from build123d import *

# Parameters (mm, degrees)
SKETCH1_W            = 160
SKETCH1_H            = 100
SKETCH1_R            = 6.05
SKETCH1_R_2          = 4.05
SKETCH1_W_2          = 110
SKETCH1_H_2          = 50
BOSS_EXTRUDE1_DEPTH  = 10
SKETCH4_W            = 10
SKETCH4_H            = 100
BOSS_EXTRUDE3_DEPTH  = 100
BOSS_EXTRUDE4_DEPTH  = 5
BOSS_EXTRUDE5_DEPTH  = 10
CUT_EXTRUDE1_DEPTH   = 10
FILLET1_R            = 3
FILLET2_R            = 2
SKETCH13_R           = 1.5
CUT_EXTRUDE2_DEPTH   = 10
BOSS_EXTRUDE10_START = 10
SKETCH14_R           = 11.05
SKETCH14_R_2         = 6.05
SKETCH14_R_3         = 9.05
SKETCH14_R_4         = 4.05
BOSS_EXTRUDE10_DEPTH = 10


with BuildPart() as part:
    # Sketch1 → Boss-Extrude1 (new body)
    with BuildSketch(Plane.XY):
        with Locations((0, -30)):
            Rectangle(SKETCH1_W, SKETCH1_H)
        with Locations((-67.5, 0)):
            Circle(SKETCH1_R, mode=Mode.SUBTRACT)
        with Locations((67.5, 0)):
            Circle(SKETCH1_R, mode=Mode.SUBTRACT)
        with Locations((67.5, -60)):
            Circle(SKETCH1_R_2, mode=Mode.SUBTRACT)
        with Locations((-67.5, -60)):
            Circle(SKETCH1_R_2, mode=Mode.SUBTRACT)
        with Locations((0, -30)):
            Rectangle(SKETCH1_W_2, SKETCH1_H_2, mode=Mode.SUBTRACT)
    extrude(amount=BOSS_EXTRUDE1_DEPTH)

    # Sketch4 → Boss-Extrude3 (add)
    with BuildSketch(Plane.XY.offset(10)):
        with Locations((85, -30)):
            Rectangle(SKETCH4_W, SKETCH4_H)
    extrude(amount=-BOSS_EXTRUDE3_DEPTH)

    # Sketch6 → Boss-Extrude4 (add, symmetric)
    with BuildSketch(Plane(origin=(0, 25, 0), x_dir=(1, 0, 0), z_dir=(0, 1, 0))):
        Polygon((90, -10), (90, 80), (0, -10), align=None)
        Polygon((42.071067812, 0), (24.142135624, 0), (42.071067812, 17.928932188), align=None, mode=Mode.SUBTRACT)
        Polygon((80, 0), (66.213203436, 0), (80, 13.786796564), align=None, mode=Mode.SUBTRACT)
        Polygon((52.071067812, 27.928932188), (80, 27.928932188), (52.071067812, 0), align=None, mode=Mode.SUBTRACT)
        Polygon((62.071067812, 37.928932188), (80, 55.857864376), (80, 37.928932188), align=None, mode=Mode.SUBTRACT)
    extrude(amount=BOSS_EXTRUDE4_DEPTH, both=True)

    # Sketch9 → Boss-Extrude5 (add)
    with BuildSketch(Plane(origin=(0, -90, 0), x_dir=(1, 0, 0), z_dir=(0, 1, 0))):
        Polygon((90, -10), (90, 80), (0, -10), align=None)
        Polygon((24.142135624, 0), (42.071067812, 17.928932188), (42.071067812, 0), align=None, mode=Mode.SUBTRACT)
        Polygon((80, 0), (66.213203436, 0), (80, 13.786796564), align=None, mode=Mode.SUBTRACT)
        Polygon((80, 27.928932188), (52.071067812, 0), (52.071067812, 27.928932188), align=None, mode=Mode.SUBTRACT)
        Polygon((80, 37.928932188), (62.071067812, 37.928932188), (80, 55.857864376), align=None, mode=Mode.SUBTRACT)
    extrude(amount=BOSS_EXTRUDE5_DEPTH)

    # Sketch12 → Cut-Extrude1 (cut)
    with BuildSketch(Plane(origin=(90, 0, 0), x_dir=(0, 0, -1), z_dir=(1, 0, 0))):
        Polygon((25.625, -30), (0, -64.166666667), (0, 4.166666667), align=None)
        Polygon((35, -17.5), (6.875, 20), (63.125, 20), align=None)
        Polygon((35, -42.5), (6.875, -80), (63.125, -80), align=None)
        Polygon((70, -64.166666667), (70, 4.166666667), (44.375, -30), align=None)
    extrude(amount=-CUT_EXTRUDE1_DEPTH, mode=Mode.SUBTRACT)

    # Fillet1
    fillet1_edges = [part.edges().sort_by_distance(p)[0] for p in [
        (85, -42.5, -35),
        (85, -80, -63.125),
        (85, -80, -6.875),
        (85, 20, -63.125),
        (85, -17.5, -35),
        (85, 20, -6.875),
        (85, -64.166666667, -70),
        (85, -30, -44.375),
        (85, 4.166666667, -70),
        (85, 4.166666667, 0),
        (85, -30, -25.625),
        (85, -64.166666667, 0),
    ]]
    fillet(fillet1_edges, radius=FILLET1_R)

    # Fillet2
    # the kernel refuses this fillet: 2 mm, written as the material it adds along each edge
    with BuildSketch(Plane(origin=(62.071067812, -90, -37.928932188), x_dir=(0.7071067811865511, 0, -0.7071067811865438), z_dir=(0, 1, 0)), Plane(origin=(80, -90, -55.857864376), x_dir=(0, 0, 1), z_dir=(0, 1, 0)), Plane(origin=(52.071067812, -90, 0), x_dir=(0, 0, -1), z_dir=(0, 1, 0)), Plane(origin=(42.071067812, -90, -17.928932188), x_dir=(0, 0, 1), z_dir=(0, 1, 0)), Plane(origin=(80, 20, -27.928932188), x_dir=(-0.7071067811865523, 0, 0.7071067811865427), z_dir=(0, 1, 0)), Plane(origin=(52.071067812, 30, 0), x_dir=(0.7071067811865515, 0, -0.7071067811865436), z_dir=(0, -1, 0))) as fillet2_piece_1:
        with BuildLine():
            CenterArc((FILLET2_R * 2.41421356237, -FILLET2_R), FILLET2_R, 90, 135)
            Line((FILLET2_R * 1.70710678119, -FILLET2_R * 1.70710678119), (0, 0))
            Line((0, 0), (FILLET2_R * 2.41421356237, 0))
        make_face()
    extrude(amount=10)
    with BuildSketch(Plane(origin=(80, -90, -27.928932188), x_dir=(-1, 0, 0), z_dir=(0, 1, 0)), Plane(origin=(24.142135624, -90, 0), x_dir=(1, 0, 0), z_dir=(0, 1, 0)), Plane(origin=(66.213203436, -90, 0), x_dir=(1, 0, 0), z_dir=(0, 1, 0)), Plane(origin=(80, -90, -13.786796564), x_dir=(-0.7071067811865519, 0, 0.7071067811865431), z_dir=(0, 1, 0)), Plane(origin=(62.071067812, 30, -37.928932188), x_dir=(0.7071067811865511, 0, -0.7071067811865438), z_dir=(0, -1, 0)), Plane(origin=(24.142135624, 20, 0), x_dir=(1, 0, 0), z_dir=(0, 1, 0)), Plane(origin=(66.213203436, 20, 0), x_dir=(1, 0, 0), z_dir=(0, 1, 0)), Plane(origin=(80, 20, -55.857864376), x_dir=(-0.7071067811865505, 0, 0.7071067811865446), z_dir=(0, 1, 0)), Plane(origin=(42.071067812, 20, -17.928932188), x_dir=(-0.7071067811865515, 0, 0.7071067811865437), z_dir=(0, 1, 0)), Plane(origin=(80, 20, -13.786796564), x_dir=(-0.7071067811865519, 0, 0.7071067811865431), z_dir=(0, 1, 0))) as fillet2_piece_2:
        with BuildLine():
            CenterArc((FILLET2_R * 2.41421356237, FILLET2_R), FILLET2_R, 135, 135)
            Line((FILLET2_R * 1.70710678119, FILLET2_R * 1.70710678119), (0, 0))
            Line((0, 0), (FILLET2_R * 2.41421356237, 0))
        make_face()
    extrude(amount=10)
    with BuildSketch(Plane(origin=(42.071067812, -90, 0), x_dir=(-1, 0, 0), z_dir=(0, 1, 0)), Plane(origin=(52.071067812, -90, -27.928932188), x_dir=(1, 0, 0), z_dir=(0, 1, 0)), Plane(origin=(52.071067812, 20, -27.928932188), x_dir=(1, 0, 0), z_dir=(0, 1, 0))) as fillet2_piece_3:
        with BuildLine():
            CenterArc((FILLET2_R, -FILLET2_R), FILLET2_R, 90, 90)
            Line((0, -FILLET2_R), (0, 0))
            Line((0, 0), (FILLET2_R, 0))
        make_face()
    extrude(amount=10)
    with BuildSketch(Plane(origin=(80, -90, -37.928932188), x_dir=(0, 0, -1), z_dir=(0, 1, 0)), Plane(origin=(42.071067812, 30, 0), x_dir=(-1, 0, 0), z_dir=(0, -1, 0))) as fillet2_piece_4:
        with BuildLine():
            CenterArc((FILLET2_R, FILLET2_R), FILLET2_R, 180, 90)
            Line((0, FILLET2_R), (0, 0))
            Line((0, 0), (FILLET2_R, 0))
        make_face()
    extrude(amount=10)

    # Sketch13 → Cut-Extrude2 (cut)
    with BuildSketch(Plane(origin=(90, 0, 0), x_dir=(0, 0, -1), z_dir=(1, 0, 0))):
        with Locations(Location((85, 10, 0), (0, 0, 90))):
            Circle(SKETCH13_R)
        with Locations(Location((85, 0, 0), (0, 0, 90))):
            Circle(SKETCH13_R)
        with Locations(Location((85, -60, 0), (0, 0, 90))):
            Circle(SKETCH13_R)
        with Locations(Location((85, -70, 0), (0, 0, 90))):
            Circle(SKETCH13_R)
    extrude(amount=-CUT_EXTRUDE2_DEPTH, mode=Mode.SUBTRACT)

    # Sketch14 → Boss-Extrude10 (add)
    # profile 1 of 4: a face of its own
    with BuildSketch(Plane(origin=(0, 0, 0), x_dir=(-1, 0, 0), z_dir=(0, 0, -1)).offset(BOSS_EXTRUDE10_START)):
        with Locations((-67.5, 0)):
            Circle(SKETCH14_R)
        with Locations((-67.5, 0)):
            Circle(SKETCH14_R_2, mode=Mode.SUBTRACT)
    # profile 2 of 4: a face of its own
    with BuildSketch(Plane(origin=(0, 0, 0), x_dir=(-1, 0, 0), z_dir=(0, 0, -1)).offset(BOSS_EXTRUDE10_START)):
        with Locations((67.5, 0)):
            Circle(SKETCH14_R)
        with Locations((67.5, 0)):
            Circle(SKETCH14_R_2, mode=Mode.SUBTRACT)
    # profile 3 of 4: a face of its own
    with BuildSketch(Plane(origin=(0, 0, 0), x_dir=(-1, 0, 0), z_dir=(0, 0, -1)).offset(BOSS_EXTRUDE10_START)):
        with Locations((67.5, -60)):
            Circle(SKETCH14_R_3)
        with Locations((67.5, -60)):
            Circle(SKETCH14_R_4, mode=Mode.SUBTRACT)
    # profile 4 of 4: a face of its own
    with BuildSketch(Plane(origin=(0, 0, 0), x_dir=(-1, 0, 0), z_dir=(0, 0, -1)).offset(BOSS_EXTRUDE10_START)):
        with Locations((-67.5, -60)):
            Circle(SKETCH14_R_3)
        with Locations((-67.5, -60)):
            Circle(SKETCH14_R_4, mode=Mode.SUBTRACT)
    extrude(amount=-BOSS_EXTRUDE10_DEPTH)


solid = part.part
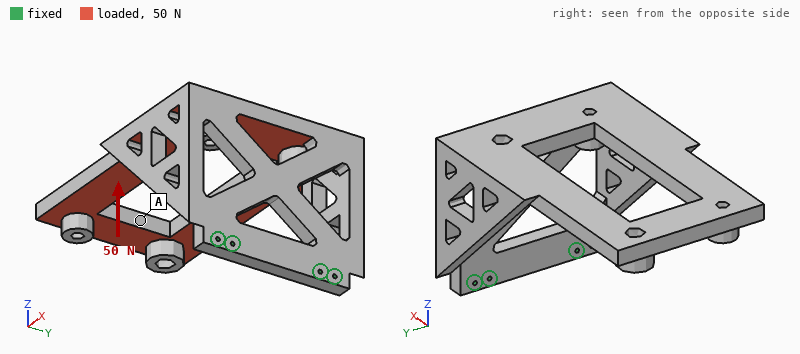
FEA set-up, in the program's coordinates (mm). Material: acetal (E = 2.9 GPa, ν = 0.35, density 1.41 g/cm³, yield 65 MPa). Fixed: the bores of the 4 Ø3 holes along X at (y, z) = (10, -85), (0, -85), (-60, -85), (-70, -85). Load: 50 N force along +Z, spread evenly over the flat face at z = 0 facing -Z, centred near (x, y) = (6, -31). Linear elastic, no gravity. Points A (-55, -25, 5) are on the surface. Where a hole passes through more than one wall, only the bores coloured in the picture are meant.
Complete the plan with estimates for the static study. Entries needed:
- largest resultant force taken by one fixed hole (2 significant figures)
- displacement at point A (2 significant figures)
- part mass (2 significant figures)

38 N
2.0 mm
340 g
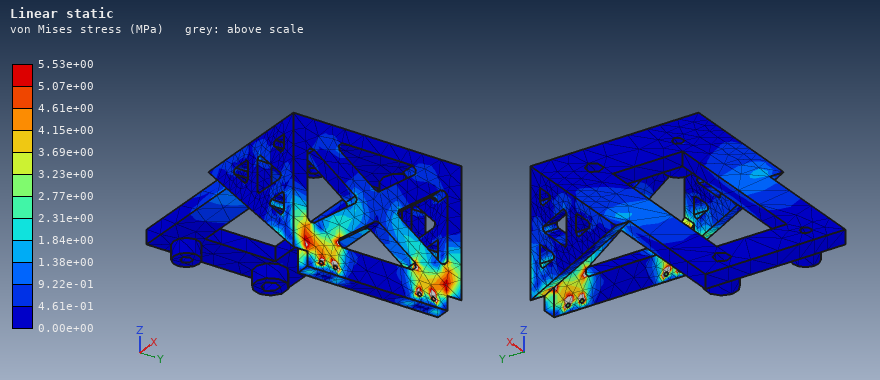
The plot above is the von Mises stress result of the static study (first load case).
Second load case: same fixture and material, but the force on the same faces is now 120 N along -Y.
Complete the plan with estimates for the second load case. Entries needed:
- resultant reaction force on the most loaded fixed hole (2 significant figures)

180 N
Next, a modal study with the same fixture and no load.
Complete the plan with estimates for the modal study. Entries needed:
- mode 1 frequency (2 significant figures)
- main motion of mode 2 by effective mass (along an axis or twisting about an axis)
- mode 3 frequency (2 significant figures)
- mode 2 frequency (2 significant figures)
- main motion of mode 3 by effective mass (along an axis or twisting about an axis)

54 Hz
along Y
200 Hz
96 Hz
along X
